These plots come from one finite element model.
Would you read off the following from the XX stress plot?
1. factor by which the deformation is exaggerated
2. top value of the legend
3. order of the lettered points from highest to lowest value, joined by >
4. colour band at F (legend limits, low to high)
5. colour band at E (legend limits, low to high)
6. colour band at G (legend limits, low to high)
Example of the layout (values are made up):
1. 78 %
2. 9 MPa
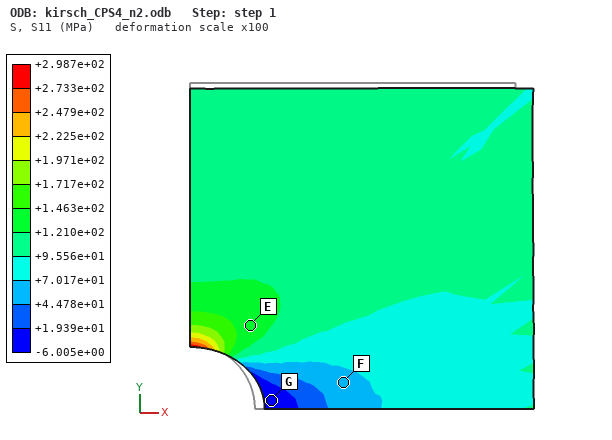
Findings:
1. 100
2. +2.987e+02 MPa
3. E > F > G
4. +4.478e+01 to +7.017e+01 MPa
5. +1.210e+02 to +1.463e+02 MPa
6. -6.005e+00 to +1.939e+01 MPa
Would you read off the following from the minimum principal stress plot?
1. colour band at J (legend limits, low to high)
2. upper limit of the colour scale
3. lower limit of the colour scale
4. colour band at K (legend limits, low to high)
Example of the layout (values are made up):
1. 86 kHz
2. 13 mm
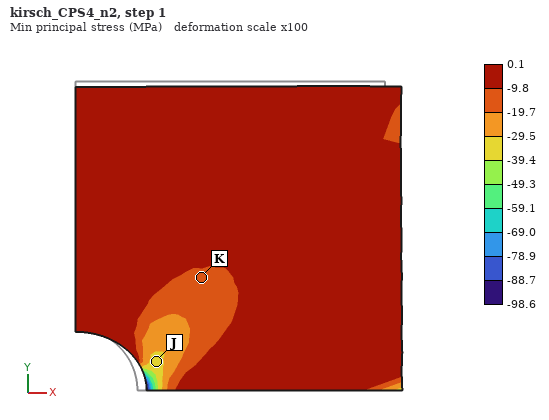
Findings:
1. -39.4 to -29.5 MPa
2. 0.1 MPa
3. -98.6 MPa
4. -19.7 to -9.8 MPa
